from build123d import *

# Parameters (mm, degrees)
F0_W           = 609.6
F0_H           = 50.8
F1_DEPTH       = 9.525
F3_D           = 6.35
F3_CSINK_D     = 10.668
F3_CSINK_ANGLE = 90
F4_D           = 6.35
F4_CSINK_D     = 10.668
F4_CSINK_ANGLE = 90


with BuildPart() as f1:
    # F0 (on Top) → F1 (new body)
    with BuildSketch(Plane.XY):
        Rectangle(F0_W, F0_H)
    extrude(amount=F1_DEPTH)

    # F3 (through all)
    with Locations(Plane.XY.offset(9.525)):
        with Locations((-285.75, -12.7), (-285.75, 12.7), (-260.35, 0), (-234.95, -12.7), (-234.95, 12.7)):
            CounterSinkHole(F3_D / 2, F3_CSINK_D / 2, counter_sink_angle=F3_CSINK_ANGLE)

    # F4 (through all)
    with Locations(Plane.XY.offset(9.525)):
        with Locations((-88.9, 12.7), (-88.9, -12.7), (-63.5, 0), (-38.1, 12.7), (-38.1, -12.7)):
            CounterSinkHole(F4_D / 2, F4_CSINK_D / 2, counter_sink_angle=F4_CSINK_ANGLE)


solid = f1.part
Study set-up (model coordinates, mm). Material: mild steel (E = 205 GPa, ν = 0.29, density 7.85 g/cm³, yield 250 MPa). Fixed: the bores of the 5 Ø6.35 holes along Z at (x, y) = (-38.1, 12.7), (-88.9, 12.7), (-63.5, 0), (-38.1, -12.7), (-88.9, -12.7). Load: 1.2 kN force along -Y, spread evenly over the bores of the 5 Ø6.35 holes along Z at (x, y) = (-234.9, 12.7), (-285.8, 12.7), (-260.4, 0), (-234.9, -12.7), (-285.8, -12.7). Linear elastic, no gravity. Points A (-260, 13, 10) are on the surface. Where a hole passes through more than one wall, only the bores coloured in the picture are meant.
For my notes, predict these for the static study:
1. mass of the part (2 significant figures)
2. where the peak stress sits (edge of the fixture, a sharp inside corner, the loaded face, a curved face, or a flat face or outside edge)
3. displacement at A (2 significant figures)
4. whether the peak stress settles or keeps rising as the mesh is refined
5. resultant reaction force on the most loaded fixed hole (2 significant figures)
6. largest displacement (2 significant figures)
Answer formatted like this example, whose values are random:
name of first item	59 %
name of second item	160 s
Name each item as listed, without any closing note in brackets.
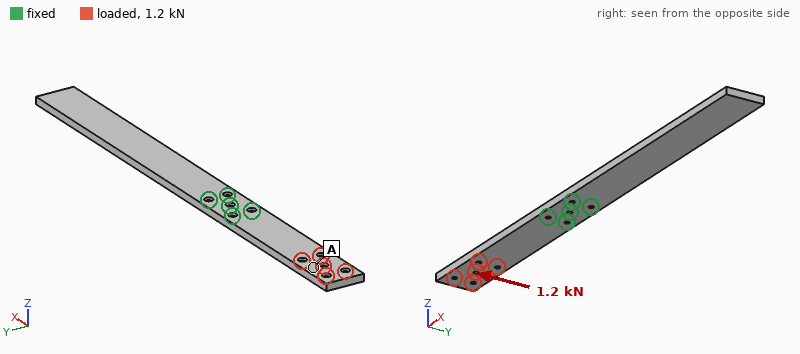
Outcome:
mass of the part	2.3 kg
where the peak stress sits	edge of the fixture
displacement at A	0.11 mm
whether the peak stress settles or keeps rising as the mesh is refined	keeps rising
resultant reaction force on the most loaded fixed hole	5.6 kN
largest displacement	0.15 mm
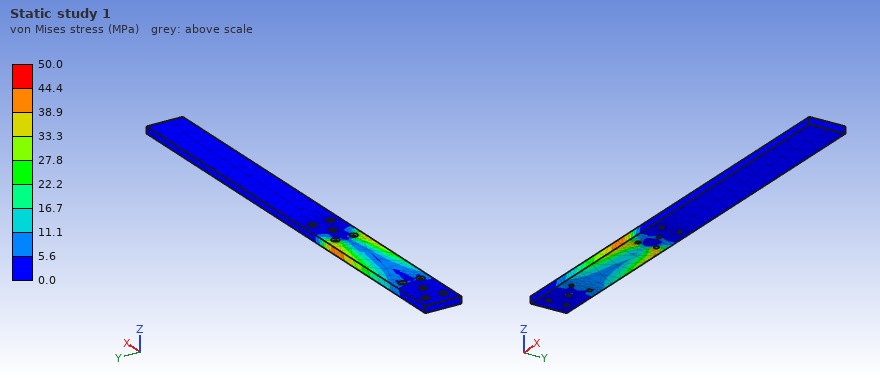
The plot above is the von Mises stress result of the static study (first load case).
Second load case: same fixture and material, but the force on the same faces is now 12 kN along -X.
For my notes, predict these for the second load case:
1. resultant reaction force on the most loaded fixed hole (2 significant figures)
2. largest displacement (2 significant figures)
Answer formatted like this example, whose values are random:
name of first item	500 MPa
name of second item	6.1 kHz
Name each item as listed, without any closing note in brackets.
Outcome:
resultant reaction force on the most loaded fixed hole	5.3 kN
largest displacement	0.38 mm
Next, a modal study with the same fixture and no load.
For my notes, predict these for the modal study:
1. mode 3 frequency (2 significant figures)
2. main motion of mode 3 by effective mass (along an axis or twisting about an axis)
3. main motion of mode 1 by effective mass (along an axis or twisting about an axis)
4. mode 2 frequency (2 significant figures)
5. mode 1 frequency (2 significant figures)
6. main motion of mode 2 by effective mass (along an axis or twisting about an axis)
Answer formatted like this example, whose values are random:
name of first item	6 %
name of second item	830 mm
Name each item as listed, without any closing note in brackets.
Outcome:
mode 3 frequency	340 Hz
main motion of mode 3 by effective mass	along Y
main motion of mode 1 by effective mass	along Z
mode 2 frequency	170 Hz
mode 1 frequency	66 Hz
main motion of mode 2 by effective mass	along Z
